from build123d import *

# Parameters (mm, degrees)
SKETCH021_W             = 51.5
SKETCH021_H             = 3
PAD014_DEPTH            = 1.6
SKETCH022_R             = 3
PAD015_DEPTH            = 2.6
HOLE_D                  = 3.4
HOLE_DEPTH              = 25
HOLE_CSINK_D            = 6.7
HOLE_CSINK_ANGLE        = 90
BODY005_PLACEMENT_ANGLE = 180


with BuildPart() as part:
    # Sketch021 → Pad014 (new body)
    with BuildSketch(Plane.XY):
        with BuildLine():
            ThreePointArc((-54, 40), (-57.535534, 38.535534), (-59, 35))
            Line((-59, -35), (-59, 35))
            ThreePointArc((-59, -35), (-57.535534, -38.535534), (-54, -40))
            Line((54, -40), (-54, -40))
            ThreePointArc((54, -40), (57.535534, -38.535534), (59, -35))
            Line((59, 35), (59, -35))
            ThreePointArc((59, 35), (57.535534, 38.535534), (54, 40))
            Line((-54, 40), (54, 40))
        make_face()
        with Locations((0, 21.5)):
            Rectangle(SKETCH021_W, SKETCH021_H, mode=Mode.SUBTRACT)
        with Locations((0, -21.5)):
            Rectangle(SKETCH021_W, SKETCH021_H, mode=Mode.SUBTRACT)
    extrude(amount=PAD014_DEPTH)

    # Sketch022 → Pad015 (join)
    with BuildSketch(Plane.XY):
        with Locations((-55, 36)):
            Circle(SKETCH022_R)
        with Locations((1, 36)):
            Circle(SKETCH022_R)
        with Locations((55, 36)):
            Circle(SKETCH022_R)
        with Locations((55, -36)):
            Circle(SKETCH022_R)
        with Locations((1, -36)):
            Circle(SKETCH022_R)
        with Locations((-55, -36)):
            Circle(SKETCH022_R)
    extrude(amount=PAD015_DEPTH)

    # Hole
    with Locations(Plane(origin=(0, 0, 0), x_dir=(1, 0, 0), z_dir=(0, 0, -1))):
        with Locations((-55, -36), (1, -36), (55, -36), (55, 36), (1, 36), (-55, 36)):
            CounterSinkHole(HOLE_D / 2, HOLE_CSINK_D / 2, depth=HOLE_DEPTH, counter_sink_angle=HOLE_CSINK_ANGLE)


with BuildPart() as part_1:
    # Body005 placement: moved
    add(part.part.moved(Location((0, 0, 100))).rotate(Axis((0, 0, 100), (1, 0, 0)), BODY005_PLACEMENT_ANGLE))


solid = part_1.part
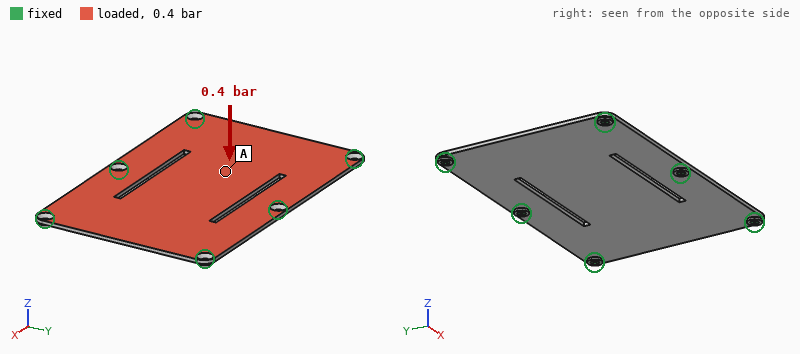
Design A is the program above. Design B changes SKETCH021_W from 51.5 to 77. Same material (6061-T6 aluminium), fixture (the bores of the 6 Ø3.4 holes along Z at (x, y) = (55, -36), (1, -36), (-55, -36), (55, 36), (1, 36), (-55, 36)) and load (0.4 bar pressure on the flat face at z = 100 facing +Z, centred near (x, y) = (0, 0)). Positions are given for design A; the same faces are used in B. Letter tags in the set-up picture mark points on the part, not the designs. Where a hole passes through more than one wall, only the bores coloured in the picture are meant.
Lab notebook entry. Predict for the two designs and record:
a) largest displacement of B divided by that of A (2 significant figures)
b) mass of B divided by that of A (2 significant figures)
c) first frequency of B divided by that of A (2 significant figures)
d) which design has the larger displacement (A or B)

1.9
0.98
0.71
B
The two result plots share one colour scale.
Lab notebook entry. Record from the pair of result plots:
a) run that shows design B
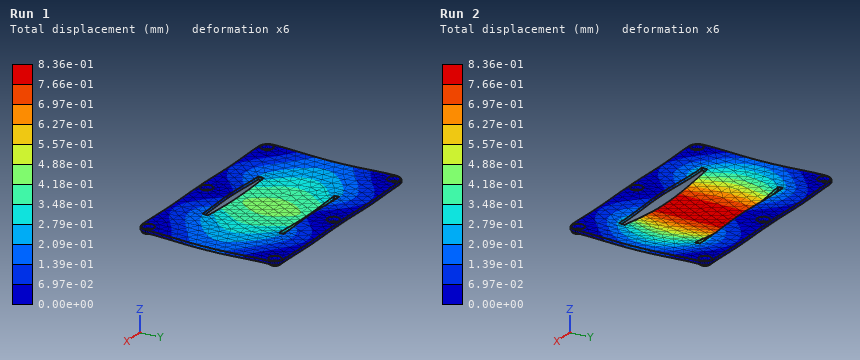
Run 2
